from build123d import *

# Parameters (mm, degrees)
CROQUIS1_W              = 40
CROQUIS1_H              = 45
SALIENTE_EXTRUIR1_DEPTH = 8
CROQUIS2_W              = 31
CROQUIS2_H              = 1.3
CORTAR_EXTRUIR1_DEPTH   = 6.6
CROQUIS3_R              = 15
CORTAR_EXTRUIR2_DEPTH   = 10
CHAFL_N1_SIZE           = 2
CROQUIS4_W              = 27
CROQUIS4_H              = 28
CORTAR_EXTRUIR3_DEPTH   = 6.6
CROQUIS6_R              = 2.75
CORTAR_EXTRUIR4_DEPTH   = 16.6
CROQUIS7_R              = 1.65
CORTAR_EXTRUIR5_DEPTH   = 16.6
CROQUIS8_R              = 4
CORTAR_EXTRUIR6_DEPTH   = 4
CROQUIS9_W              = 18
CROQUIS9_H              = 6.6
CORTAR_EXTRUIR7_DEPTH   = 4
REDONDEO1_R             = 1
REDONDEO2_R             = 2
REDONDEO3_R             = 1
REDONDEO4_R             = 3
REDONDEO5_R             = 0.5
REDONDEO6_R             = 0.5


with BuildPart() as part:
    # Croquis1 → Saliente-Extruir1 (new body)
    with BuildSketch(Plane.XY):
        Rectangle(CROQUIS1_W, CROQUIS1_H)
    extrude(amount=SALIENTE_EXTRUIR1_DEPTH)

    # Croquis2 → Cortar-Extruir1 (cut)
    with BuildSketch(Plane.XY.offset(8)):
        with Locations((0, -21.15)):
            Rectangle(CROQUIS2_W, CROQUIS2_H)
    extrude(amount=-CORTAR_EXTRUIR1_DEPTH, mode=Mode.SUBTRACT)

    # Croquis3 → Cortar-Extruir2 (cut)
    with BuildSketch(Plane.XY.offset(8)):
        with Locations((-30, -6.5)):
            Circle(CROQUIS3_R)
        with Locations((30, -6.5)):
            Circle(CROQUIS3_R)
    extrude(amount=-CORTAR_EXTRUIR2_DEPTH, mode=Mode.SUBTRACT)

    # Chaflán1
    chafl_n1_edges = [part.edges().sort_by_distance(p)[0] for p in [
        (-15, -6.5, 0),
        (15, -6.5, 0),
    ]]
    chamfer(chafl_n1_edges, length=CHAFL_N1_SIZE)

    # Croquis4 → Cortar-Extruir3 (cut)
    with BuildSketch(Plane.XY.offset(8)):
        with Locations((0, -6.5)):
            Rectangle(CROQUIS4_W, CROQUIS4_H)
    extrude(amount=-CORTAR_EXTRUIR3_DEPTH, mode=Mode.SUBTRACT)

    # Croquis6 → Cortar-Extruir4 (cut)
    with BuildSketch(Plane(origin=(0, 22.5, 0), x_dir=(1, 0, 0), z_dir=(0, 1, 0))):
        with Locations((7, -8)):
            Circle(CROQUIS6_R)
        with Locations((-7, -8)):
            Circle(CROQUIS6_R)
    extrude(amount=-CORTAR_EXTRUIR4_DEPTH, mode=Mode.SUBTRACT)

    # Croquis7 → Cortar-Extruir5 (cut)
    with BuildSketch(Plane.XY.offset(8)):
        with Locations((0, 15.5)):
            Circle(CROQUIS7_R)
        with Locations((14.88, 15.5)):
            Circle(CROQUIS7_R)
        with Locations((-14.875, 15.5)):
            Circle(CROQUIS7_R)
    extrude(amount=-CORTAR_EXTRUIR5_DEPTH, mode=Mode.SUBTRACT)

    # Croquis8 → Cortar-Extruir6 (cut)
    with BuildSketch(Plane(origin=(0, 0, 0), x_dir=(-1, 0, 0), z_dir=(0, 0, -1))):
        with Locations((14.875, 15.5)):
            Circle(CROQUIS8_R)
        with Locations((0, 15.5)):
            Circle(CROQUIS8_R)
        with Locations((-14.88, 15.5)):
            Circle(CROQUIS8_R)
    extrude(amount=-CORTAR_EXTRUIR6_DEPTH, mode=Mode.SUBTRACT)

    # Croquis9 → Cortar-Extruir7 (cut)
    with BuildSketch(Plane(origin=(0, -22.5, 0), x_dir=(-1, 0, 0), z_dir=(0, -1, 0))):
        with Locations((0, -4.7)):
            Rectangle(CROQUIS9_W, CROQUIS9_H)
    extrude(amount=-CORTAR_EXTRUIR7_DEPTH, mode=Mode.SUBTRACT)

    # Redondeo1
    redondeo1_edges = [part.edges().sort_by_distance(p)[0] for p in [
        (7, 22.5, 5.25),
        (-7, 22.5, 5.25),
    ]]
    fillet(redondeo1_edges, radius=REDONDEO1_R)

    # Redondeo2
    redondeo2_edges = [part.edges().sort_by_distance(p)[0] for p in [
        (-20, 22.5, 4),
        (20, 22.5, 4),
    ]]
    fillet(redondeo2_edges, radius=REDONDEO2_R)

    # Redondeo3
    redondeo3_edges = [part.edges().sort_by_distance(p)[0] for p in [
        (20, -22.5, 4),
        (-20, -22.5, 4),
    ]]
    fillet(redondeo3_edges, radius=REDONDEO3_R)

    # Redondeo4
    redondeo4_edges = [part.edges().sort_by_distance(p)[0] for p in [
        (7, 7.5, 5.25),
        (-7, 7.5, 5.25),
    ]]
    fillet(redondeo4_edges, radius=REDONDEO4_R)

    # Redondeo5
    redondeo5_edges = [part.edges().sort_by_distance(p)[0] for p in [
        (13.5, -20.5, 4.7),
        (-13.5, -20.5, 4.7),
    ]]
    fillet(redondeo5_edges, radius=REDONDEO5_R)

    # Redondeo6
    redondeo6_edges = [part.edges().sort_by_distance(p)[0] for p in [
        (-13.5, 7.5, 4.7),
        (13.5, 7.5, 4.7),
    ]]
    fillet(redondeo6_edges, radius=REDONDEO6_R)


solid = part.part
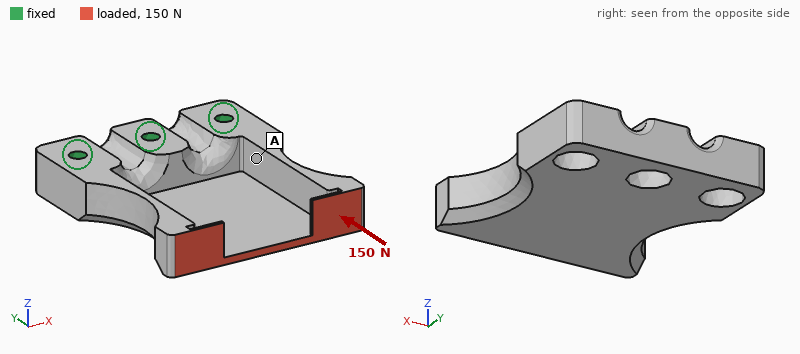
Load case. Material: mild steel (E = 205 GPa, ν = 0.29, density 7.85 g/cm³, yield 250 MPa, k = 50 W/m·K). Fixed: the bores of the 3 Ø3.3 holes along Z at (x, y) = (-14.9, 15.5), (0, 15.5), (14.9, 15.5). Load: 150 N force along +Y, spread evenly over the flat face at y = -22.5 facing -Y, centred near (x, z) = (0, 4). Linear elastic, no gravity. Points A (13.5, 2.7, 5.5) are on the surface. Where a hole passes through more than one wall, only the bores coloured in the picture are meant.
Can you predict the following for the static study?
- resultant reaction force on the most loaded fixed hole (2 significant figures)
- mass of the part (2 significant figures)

61 N
52 g
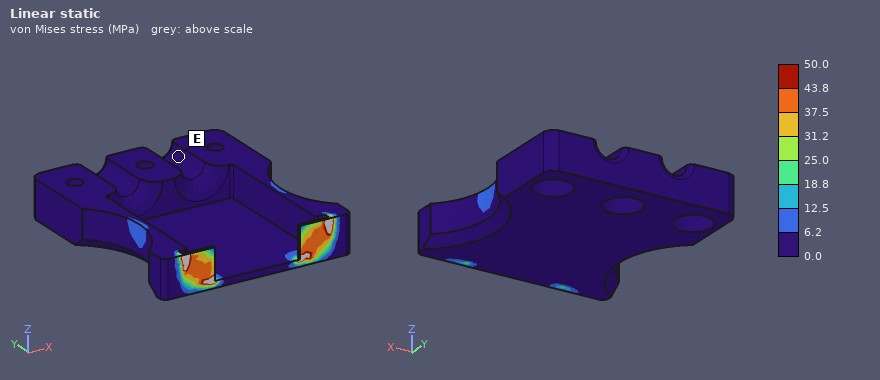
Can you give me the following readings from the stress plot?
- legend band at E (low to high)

0.0 to 6.2 MPa
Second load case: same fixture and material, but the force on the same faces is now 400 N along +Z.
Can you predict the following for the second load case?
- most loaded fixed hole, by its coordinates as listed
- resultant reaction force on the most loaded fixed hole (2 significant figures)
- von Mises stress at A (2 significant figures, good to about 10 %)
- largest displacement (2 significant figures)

(0, 15.5)
760 N
64 MPa
0.11 mm
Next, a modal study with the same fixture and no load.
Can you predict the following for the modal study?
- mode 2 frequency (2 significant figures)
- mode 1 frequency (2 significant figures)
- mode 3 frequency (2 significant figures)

3700 Hz
3700 Hz
5600 Hz
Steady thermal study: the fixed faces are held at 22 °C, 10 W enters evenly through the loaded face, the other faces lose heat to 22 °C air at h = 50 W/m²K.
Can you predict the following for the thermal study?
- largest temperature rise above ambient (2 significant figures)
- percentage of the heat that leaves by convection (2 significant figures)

78 K
48 %
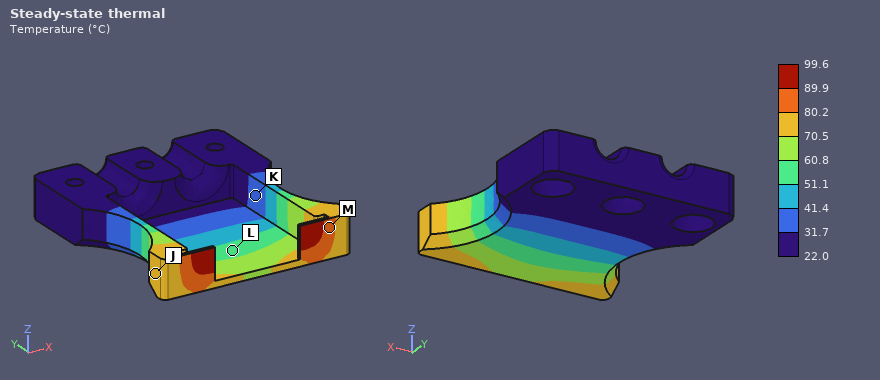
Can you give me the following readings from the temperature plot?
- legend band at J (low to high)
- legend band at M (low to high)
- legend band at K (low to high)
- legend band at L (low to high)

70.5 to 80.2 °C
80.2 to 89.9 °C
31.7 to 41.4 °C
51.1 to 60.8 °C
